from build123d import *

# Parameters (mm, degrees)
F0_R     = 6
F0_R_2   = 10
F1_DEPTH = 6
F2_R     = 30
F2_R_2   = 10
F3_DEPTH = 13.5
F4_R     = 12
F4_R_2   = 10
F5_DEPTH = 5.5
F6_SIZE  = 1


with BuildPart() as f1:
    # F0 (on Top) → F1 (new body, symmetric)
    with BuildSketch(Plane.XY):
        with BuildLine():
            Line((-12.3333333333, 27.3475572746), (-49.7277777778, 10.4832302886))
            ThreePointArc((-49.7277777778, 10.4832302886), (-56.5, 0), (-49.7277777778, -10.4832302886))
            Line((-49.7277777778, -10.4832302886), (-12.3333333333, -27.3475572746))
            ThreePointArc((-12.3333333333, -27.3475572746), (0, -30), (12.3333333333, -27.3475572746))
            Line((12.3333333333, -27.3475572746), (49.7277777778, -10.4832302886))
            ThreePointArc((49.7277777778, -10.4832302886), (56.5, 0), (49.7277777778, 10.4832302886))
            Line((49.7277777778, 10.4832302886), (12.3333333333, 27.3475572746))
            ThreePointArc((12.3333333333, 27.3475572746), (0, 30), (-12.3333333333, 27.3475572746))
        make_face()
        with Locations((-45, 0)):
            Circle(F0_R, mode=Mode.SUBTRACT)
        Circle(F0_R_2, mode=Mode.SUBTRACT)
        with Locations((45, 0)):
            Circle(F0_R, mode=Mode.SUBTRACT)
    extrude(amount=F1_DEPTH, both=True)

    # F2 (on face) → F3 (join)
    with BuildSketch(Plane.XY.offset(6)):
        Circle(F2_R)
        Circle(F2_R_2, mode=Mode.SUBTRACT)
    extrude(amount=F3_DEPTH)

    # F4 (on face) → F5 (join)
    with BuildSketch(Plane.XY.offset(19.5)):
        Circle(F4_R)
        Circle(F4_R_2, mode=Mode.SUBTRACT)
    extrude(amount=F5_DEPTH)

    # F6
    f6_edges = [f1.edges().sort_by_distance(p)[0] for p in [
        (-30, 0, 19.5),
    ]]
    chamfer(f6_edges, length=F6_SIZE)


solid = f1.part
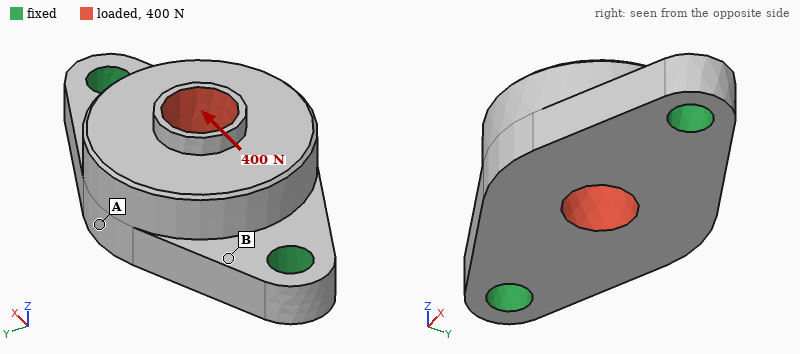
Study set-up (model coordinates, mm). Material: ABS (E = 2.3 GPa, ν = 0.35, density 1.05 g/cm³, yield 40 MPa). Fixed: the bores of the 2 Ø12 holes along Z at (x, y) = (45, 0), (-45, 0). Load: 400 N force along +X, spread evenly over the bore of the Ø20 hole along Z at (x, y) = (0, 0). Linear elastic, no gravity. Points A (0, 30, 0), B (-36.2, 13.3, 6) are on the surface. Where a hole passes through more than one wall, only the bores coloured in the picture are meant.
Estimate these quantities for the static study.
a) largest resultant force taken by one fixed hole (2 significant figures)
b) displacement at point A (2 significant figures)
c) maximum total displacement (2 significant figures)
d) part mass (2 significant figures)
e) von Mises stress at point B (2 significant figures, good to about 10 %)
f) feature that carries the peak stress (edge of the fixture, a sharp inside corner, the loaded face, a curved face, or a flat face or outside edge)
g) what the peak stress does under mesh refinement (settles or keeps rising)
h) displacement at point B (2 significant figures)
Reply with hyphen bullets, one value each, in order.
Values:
- 210 N
- 4.9 µm
- 19 µm
- 86 g
- 0.40 MPa
- edge of the fixture
- keeps rising
- 3.5 µm
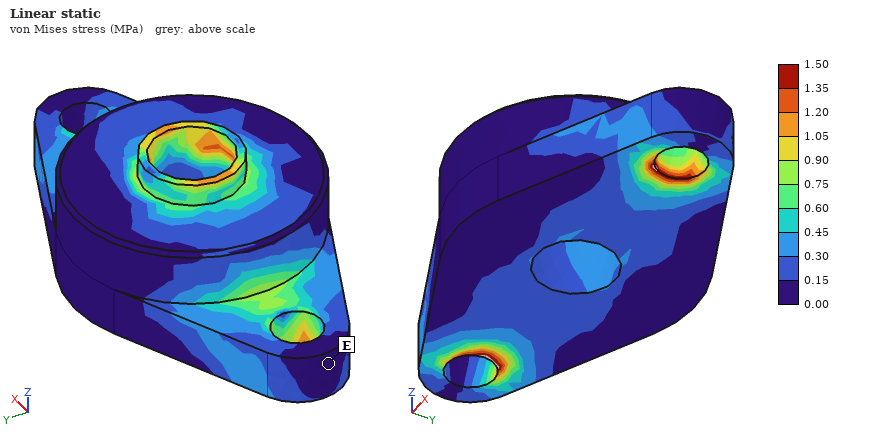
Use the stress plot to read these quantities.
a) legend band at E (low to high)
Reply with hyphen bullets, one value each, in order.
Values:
- 0.00 to 0.15 MPa
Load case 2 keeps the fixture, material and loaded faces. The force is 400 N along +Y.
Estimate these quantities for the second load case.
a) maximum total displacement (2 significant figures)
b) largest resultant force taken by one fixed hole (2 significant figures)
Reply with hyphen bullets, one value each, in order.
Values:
- 86 µm
- 200 N
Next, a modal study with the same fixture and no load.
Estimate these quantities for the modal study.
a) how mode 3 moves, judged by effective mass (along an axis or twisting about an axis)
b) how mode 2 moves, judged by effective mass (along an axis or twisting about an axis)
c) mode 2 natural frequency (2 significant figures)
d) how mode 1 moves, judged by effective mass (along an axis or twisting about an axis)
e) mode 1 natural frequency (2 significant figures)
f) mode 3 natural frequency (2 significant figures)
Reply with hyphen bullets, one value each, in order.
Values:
- along Y
- along Z
- 2100 Hz
- along Y
- 1300 Hz
- 3100 Hz
